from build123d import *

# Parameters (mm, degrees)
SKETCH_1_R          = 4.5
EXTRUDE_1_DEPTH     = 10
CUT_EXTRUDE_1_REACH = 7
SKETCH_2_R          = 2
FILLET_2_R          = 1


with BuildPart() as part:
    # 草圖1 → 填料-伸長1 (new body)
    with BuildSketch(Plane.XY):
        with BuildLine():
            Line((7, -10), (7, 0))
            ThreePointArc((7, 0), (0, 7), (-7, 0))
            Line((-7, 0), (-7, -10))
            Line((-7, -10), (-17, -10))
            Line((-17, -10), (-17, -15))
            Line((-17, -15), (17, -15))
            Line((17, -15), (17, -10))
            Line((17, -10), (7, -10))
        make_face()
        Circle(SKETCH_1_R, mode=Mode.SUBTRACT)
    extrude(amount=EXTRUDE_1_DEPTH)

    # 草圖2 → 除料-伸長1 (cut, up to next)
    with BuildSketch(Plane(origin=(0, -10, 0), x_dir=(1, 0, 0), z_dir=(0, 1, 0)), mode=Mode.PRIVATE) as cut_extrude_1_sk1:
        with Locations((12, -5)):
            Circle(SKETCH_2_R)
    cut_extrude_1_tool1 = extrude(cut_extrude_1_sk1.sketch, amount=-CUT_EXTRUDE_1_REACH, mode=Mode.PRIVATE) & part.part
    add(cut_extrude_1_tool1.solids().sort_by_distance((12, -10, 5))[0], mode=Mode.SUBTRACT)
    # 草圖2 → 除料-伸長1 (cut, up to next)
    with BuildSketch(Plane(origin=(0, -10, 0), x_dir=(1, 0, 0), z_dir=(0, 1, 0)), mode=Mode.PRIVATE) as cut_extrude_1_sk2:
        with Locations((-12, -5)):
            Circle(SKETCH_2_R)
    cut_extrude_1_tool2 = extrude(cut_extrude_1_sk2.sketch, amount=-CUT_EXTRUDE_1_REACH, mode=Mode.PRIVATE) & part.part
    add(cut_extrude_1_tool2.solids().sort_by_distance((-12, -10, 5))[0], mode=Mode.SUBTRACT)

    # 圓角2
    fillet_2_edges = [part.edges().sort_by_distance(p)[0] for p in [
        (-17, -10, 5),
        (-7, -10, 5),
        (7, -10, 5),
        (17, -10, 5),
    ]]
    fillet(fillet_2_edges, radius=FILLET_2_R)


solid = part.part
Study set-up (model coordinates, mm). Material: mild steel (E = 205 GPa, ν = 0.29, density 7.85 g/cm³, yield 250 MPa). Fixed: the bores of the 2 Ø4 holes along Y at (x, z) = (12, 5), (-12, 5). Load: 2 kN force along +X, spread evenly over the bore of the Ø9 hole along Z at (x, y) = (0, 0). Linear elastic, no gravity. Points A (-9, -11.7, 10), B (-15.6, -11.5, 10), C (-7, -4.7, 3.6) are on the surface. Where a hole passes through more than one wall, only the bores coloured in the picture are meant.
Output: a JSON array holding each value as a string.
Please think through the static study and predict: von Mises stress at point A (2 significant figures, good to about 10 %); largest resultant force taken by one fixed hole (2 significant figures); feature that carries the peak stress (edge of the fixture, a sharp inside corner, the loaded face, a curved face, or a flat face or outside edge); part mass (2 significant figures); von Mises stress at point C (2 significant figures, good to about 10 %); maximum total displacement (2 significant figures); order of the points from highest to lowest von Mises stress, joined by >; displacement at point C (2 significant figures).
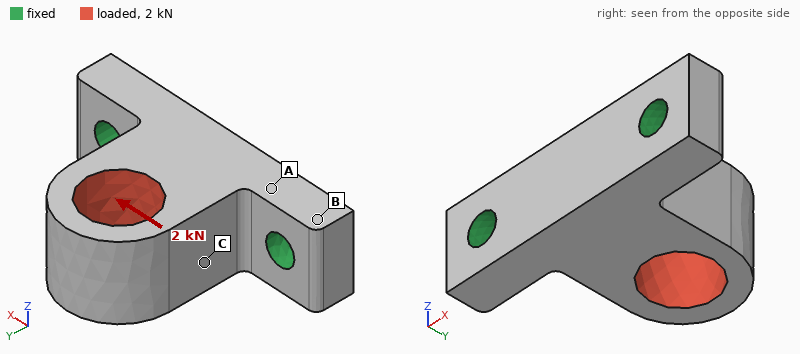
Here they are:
["54 MPa", "1.7 kN", "a curved face", "24 g", "92 MPa", "22 µm", "C > A > B", "6.6 µm"]
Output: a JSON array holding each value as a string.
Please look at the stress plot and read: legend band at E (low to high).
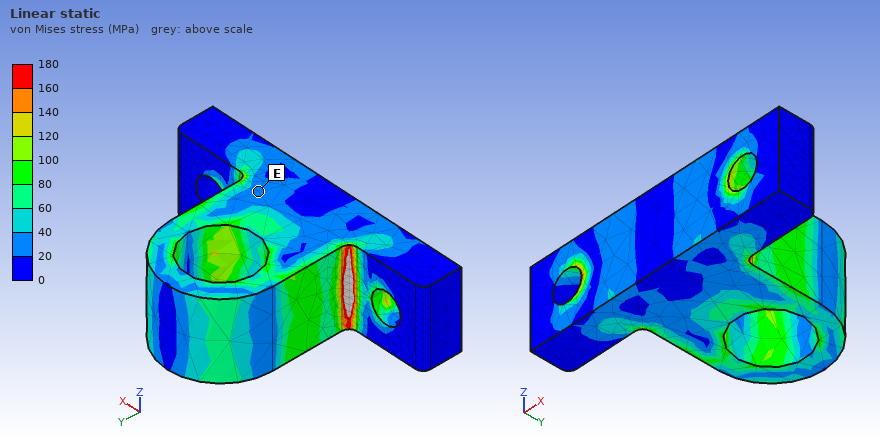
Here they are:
["20 to 40 MPa"]
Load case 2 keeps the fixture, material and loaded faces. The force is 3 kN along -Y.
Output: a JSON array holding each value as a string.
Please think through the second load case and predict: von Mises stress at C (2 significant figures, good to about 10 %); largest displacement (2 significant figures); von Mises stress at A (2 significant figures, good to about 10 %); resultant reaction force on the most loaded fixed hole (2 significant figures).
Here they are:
["47 MPa", "8.1 µm", "51 MPa", "1.6 kN"]
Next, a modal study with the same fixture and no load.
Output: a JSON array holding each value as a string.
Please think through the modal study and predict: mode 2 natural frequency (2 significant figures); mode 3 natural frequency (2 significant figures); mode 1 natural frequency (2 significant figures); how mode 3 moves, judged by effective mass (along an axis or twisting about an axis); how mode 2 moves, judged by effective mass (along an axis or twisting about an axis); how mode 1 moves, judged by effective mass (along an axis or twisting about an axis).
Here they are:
["20 kHz", "31 kHz", "11 kHz", "along Y", "along X", "along Z"]
